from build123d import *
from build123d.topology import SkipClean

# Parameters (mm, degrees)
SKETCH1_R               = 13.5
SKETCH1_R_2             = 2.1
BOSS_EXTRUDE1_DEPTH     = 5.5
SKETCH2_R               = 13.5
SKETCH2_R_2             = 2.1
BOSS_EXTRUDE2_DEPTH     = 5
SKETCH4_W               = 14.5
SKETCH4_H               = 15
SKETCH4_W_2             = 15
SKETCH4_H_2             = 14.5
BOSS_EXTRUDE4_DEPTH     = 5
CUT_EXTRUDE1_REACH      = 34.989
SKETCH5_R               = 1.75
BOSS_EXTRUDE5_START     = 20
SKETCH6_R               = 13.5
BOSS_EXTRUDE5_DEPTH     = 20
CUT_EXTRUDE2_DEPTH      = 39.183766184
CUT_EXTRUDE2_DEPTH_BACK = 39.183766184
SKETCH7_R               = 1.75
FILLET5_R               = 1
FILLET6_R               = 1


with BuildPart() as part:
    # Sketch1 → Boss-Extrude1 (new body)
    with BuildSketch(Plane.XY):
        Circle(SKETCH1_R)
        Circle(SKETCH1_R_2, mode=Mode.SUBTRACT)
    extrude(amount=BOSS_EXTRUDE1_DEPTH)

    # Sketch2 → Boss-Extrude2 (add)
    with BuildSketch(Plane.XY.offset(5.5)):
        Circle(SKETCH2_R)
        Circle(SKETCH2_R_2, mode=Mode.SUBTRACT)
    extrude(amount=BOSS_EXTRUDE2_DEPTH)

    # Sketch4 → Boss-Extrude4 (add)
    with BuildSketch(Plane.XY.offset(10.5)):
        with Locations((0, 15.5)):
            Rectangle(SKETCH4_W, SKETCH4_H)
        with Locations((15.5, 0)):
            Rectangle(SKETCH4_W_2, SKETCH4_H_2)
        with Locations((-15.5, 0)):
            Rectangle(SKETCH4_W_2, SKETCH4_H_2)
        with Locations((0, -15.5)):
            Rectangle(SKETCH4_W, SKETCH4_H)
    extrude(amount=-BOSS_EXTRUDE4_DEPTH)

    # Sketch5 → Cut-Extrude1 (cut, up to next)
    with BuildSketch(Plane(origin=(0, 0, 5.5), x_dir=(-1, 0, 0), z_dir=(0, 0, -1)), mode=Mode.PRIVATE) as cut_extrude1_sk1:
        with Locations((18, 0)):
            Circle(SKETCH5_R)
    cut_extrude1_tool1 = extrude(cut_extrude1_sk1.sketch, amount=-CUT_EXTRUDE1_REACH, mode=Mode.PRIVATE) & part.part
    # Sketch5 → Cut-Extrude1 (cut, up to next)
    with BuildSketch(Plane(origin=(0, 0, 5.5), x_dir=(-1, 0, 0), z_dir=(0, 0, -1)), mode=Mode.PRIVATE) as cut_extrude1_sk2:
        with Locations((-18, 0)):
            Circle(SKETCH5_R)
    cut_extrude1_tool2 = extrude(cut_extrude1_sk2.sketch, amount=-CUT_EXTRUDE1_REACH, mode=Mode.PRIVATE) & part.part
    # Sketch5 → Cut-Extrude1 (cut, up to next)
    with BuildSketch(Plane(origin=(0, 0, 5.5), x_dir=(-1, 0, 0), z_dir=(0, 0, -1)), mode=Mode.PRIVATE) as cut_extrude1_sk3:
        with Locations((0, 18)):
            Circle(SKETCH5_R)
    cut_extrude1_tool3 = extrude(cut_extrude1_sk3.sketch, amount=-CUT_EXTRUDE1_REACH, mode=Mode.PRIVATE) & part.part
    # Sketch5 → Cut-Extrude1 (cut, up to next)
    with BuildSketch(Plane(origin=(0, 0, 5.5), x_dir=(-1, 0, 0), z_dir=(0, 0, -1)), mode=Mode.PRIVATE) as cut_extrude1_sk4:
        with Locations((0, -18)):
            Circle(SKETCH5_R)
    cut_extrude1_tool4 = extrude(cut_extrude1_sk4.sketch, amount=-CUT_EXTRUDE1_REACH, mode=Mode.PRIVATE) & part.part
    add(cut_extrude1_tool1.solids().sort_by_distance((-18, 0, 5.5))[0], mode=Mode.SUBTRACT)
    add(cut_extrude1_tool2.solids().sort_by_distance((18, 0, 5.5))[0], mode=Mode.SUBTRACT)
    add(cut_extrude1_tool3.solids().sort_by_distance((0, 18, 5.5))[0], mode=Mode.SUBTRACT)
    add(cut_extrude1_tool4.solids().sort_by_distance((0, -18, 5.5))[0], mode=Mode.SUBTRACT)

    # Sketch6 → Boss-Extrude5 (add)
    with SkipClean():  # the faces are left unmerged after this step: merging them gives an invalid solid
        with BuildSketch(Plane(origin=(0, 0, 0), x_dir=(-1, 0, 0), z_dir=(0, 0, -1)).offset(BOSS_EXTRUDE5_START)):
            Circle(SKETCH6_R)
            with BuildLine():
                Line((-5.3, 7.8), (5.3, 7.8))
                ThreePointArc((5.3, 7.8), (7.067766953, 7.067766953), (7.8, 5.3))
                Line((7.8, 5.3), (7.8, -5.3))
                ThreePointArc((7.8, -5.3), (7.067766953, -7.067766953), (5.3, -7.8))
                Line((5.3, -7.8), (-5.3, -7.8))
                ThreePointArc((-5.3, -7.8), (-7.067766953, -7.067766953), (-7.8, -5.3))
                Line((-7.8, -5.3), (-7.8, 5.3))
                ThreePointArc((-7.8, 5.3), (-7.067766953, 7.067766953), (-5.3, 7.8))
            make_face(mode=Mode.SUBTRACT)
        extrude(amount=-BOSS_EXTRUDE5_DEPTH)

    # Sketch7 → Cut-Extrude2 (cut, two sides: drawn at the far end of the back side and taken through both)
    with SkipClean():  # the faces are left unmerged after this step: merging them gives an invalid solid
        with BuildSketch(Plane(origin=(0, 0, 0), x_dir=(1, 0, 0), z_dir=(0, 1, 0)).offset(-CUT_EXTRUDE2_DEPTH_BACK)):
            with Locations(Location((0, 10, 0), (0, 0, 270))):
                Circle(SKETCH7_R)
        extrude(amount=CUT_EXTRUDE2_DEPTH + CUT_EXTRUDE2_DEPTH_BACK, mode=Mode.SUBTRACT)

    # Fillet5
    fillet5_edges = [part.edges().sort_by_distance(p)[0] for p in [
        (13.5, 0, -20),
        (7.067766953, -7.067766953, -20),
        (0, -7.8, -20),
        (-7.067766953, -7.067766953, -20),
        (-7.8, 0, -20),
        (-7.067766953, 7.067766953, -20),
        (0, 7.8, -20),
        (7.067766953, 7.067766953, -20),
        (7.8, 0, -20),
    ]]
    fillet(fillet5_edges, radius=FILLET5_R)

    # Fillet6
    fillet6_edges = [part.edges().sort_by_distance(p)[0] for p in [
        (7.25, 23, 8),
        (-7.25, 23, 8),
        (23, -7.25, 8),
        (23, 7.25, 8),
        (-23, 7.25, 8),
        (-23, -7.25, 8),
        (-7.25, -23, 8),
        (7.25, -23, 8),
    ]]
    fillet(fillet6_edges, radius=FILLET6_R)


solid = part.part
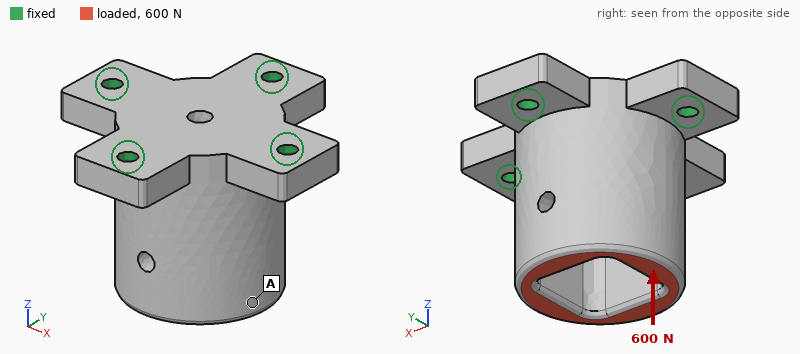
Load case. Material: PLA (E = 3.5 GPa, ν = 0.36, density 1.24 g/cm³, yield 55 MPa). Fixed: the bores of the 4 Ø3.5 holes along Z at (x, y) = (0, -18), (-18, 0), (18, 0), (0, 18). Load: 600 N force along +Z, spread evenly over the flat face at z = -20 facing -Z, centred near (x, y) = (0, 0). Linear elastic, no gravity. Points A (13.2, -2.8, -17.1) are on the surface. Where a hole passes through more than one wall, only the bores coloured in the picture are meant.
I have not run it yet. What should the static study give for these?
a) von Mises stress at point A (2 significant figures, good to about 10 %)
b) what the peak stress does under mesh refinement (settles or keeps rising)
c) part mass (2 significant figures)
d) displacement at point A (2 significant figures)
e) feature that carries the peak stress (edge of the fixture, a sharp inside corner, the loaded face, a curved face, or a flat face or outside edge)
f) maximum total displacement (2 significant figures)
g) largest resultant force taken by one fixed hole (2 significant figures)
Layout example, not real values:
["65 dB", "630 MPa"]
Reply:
["1.5 MPa", "keeps rising", "19 g", "32 µm", "edge of the fixture", "36 µm", "160 N"]
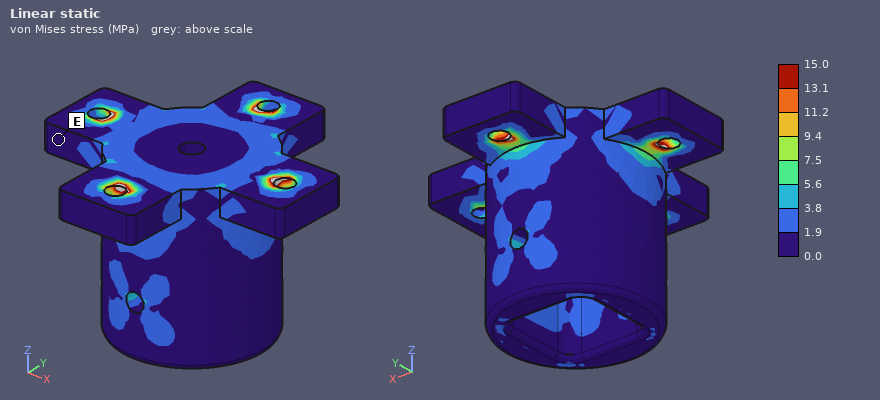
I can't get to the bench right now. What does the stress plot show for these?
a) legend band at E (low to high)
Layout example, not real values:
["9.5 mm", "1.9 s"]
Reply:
["0.0 to 1.9 MPa"]
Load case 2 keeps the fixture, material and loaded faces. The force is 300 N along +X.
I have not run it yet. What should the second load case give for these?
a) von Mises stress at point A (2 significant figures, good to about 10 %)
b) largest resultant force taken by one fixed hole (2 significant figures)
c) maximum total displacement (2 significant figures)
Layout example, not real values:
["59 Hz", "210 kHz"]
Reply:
["3.5 MPa", "290 N", "0.15 mm"]
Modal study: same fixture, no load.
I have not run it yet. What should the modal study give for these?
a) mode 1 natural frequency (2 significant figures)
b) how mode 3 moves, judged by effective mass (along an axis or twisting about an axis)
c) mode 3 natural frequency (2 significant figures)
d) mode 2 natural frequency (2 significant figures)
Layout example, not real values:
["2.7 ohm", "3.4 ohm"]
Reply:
["3900 Hz", "along Z", "6300 Hz", "3900 Hz"]
